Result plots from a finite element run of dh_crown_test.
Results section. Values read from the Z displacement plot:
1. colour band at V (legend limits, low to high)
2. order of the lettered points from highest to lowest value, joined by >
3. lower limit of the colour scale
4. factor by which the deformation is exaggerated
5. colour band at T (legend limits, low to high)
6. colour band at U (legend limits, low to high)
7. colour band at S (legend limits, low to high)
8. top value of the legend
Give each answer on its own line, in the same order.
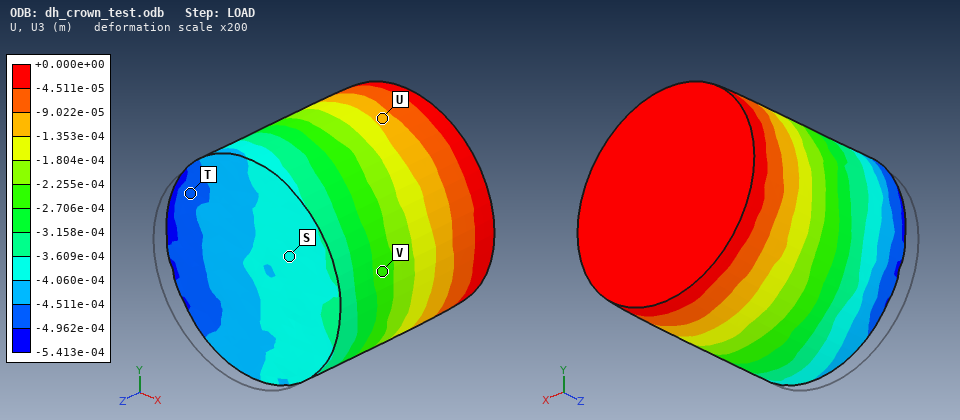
-2.706e-04 to -2.255e-04 m
U > V > S > T
-5.413e-04 m
200
-4.962e-04 to -4.511e-04 m
-1.353e-04 to -9.022e-05 m
-4.060e-04 to -3.609e-04 m
+0.000e+00 m
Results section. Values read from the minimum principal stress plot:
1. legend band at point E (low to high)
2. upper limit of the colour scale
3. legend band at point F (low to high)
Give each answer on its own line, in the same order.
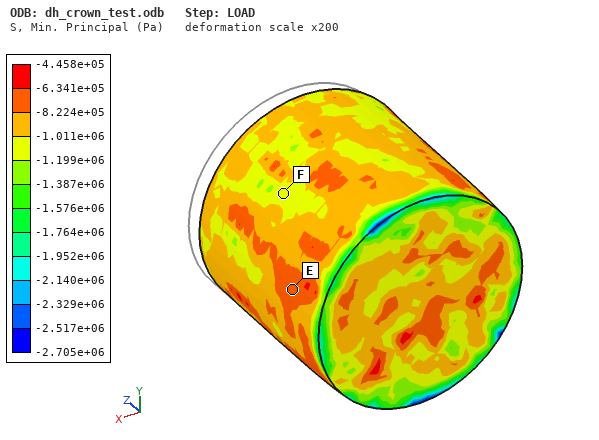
-8.224e+05 to -6.341e+05 Pa
-4.458e+05 Pa
-1.199e+06 to -1.011e+06 Pa
